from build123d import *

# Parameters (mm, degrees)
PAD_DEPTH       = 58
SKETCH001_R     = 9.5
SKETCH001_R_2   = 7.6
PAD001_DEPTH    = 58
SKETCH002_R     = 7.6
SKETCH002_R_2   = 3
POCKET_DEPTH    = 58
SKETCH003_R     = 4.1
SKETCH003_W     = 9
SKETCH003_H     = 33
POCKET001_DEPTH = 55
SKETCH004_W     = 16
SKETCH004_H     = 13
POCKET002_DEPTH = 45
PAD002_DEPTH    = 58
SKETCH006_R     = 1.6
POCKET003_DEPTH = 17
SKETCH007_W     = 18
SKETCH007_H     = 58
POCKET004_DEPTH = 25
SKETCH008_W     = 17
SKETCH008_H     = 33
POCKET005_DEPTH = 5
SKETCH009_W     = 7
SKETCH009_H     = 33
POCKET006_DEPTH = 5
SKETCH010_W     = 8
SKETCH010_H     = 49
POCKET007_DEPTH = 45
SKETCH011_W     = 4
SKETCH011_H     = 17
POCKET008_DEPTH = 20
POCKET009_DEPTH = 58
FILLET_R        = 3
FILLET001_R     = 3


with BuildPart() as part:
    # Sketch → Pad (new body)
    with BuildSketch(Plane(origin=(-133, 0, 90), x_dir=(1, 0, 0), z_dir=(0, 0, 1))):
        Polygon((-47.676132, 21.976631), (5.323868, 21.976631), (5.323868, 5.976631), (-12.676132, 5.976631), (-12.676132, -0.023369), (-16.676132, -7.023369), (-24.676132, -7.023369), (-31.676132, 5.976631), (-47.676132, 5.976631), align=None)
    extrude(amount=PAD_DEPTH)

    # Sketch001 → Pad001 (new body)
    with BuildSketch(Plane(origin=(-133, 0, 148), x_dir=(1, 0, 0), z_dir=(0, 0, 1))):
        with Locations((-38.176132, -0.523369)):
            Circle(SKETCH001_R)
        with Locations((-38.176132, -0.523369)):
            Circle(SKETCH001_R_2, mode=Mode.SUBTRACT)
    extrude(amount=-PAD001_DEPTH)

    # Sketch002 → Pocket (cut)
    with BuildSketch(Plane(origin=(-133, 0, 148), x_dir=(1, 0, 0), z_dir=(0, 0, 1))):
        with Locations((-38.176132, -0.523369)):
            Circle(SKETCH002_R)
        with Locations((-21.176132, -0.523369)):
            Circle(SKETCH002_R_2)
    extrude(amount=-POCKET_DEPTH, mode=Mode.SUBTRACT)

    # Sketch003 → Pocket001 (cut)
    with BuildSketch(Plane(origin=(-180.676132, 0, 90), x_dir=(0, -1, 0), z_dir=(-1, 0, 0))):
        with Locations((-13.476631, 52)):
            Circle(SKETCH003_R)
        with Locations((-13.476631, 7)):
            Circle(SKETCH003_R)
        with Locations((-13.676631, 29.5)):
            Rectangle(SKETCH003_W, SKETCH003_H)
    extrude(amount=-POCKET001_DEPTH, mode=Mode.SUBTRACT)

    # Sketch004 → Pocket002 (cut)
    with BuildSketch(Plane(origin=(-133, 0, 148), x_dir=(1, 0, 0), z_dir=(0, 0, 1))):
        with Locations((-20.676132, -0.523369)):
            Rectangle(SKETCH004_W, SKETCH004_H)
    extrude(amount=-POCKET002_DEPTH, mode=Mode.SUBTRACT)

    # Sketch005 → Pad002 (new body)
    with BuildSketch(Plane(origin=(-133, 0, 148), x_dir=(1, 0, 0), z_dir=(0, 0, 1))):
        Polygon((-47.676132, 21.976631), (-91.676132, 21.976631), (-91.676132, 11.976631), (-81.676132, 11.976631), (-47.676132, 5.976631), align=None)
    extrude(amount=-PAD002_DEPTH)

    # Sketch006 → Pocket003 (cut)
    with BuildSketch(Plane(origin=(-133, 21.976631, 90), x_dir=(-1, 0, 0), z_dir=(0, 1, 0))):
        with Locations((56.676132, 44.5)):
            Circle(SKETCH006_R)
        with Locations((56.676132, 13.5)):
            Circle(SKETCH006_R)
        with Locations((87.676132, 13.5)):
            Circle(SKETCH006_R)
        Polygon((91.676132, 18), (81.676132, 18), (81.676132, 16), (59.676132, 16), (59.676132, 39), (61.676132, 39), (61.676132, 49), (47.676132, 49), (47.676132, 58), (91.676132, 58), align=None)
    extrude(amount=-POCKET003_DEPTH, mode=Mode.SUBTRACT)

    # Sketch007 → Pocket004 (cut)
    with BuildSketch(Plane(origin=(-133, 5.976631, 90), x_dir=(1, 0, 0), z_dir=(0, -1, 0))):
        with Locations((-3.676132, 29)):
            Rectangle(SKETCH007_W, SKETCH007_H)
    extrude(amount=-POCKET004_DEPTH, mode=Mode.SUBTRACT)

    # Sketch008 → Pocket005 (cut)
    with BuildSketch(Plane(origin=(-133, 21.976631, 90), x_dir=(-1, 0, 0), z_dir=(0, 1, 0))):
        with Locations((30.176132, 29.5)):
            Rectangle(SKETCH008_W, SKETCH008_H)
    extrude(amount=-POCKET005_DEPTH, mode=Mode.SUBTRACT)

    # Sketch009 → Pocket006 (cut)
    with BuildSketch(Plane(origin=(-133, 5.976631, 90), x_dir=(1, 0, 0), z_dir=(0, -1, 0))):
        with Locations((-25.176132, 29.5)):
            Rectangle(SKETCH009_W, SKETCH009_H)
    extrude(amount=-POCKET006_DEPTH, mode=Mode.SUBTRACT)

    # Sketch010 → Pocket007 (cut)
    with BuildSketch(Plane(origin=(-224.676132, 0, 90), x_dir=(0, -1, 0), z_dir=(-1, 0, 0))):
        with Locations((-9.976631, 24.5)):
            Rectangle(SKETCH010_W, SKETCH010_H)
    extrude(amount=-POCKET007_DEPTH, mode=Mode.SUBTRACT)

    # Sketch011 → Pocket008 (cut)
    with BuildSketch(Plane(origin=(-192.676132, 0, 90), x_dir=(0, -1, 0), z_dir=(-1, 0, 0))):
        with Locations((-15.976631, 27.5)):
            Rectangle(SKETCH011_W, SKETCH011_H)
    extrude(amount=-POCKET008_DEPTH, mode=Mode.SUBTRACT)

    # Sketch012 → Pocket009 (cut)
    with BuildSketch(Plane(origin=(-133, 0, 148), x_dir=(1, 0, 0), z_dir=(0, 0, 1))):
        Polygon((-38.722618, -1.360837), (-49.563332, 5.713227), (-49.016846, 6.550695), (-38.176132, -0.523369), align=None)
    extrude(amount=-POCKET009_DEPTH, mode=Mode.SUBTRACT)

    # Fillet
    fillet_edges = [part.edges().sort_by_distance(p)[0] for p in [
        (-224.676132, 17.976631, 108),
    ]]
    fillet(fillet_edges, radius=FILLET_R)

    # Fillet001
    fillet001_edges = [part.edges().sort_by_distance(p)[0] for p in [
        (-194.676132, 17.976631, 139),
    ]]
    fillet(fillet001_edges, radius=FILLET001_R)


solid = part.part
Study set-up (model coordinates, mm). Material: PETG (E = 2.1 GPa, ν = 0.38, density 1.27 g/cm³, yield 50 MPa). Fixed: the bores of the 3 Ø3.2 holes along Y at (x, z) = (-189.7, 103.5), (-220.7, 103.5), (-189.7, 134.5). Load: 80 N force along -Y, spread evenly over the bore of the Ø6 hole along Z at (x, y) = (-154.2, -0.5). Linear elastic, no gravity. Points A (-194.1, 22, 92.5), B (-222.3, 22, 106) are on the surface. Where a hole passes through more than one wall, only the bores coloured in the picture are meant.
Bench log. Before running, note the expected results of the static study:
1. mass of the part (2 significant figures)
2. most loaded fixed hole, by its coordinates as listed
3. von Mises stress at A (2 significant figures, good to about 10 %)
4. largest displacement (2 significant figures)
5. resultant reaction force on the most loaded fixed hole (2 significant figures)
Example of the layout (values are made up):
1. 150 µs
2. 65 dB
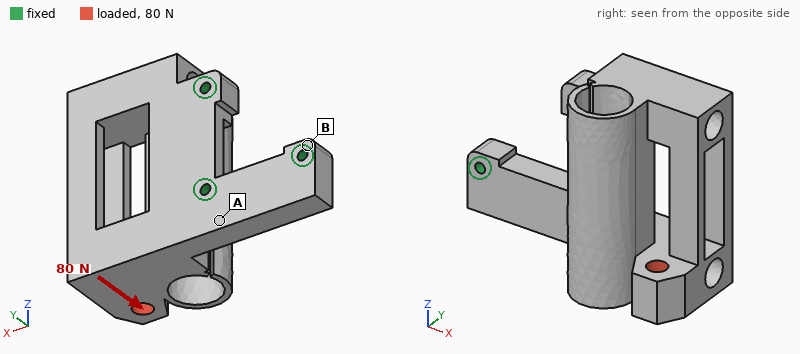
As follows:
1. 38 g
2. (-189.7, 103.5)
3. 4.3 MPa
4. 1.1 mm
5. 110 N
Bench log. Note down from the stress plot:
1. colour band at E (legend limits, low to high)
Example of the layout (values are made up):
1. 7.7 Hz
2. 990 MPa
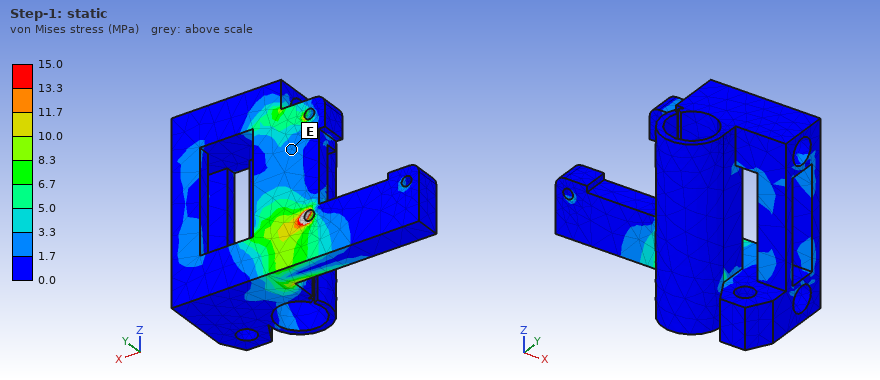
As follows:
1. 1.7 to 3.3 MPa
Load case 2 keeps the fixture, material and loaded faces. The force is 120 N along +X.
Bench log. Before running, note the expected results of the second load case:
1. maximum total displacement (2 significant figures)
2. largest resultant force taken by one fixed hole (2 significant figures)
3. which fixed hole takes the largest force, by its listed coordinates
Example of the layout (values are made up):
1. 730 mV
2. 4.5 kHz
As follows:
1. 1.1 mm
2. 92 N
3. (-189.7, 103.5)
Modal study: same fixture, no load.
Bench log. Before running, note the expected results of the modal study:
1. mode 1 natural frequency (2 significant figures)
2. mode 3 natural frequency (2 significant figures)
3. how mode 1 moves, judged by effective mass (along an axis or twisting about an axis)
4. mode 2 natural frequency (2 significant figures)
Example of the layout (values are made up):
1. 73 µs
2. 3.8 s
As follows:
1. 400 Hz
2. 630 Hz
3. along Y
4. 500 Hz
